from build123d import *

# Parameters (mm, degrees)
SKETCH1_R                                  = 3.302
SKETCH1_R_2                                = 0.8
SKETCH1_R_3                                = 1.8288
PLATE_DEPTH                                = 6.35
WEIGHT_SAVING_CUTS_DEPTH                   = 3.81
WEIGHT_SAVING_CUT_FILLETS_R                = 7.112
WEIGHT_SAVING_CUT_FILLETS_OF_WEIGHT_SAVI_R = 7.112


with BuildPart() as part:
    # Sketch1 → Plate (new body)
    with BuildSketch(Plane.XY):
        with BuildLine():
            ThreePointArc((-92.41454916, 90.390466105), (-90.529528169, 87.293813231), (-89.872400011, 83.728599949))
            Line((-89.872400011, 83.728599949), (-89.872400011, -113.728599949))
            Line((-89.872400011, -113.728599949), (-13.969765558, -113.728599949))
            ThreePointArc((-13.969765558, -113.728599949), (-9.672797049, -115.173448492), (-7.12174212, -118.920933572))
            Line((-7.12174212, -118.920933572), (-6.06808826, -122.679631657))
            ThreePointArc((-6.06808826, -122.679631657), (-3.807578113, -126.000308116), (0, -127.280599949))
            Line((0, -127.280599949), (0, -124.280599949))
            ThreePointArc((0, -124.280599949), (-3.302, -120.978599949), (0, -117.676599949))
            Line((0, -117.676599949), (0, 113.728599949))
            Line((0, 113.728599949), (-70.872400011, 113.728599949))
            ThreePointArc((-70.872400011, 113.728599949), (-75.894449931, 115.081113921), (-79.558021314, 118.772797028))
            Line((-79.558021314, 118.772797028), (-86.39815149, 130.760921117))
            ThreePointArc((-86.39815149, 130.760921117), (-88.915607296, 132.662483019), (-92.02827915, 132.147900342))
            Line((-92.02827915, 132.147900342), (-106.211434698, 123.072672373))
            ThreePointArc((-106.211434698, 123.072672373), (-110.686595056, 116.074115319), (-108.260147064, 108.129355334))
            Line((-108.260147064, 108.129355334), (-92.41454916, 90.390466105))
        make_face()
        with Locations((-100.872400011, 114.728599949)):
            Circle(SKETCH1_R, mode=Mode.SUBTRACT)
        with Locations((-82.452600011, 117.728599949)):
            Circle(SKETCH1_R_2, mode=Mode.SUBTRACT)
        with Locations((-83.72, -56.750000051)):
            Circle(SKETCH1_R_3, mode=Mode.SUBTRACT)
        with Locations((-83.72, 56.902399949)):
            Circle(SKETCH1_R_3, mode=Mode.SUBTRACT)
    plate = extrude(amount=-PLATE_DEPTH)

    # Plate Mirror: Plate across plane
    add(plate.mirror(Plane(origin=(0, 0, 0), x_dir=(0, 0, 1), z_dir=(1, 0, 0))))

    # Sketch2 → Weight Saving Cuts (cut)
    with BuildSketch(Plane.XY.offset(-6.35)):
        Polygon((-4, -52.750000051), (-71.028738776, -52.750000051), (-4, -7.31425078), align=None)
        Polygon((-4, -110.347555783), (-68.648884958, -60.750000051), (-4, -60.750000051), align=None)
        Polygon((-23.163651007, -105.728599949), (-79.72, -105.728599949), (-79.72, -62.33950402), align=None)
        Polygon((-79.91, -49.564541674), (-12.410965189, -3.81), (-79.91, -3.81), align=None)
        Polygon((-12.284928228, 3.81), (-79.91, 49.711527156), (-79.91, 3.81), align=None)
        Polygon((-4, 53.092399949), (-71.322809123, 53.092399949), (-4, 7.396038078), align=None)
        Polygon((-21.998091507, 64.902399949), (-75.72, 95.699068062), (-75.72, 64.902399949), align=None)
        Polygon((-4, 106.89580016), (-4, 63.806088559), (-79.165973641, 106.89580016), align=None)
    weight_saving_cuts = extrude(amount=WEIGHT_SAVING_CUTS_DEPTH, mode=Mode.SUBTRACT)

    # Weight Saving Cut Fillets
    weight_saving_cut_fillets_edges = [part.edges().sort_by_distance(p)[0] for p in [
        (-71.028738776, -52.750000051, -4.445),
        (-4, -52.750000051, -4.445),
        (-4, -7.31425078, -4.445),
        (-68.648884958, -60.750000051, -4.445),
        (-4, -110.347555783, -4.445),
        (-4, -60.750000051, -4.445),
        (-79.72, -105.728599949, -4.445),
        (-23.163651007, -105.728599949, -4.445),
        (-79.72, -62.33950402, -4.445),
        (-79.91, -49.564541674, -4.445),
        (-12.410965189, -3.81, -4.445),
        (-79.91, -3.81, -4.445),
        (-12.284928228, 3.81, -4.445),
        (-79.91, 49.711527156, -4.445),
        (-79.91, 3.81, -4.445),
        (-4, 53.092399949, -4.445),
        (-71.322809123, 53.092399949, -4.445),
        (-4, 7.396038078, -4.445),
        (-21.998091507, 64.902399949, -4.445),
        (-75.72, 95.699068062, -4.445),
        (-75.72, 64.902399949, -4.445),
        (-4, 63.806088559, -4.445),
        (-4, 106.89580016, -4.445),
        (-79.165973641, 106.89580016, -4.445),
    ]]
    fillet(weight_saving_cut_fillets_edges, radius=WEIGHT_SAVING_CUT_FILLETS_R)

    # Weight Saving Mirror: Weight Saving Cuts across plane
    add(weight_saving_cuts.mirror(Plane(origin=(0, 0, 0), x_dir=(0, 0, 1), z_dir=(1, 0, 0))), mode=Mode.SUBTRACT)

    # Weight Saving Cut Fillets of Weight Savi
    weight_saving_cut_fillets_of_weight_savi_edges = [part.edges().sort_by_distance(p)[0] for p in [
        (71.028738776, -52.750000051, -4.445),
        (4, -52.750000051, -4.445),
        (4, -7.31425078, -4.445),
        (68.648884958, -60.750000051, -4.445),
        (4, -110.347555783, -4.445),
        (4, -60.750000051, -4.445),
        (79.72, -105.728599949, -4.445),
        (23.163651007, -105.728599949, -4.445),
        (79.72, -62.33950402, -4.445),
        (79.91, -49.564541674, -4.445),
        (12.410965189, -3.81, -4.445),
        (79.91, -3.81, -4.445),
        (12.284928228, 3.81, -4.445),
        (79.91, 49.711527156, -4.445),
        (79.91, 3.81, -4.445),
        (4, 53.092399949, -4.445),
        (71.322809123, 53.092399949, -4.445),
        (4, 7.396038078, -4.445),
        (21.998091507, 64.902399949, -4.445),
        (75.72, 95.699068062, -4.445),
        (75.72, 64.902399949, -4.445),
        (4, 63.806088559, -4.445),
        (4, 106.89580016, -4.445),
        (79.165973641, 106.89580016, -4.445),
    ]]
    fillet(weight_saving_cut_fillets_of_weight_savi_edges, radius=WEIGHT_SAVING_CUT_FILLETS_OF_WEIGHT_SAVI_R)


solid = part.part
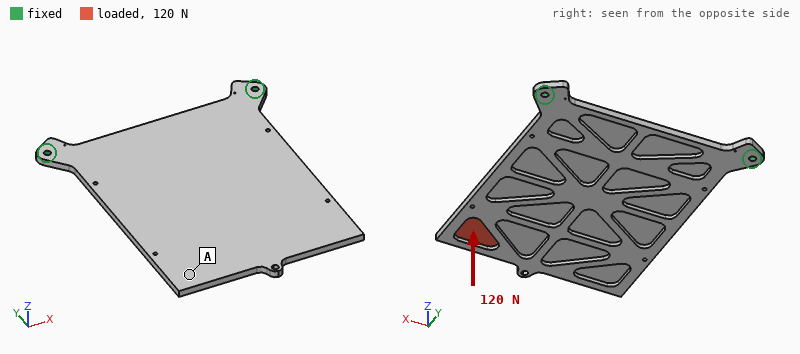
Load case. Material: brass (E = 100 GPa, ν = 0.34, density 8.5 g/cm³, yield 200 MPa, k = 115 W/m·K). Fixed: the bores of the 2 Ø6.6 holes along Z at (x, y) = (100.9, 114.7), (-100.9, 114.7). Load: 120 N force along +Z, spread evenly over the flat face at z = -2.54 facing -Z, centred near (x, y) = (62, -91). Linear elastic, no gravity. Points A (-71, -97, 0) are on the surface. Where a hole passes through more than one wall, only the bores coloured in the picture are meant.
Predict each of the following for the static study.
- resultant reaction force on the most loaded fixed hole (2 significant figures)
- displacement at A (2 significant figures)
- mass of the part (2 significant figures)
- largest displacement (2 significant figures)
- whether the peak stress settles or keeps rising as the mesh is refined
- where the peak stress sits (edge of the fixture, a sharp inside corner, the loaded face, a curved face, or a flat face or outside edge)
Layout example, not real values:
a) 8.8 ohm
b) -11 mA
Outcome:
a) 230 N
b) 2.4 mm
c) 1.6 kg
d) 3.4 mm
e) keeps rising
f) edge of the fixture
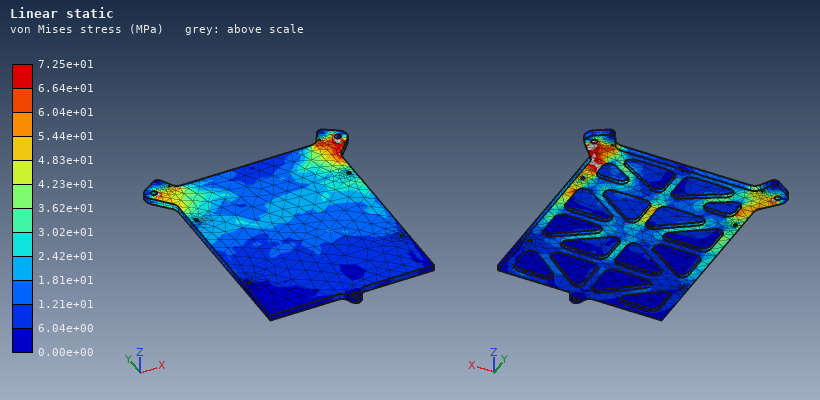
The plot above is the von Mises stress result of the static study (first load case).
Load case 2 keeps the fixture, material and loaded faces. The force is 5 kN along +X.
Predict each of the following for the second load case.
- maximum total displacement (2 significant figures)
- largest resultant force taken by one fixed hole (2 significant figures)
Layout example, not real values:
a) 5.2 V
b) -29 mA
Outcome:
a) 0.37 mm
b) 5.9 kN
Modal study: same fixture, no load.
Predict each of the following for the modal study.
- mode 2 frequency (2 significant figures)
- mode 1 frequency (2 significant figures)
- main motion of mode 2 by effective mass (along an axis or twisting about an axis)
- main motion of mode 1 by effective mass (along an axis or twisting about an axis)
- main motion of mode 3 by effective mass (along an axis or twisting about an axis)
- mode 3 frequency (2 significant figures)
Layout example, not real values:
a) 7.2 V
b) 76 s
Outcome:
a) 160 Hz
b) 46 Hz
c) twisting about Y
d) along Z
e) along Z
f) 280 Hz
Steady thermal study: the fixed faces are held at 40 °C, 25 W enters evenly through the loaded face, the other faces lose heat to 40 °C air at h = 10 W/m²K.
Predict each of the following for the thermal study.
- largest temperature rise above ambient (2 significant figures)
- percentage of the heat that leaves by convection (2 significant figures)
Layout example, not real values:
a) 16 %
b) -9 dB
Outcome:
a) 58 K
b) 72 %
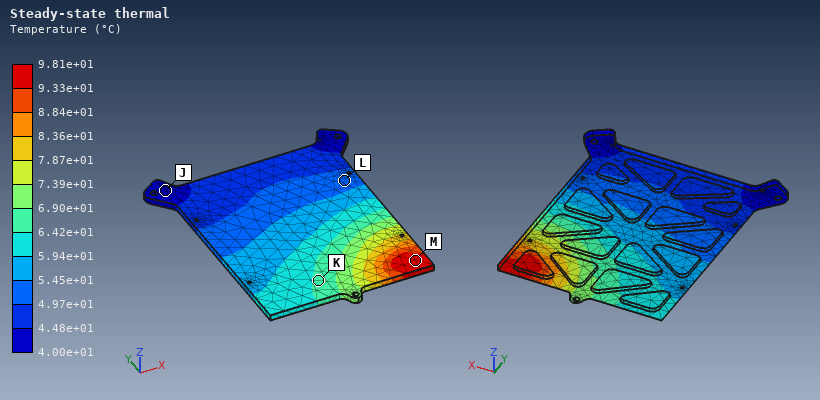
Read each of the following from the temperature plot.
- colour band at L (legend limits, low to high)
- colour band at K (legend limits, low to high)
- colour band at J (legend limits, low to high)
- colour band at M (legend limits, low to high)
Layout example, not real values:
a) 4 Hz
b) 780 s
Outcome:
a) 4.97e+01 to 5.45e+01 °C
b) 6.42e+01 to 6.90e+01 °C
c) 4.00e+01 to 4.48e+01 °C
d) 9.33e+01 to 9.81e+01 °C
